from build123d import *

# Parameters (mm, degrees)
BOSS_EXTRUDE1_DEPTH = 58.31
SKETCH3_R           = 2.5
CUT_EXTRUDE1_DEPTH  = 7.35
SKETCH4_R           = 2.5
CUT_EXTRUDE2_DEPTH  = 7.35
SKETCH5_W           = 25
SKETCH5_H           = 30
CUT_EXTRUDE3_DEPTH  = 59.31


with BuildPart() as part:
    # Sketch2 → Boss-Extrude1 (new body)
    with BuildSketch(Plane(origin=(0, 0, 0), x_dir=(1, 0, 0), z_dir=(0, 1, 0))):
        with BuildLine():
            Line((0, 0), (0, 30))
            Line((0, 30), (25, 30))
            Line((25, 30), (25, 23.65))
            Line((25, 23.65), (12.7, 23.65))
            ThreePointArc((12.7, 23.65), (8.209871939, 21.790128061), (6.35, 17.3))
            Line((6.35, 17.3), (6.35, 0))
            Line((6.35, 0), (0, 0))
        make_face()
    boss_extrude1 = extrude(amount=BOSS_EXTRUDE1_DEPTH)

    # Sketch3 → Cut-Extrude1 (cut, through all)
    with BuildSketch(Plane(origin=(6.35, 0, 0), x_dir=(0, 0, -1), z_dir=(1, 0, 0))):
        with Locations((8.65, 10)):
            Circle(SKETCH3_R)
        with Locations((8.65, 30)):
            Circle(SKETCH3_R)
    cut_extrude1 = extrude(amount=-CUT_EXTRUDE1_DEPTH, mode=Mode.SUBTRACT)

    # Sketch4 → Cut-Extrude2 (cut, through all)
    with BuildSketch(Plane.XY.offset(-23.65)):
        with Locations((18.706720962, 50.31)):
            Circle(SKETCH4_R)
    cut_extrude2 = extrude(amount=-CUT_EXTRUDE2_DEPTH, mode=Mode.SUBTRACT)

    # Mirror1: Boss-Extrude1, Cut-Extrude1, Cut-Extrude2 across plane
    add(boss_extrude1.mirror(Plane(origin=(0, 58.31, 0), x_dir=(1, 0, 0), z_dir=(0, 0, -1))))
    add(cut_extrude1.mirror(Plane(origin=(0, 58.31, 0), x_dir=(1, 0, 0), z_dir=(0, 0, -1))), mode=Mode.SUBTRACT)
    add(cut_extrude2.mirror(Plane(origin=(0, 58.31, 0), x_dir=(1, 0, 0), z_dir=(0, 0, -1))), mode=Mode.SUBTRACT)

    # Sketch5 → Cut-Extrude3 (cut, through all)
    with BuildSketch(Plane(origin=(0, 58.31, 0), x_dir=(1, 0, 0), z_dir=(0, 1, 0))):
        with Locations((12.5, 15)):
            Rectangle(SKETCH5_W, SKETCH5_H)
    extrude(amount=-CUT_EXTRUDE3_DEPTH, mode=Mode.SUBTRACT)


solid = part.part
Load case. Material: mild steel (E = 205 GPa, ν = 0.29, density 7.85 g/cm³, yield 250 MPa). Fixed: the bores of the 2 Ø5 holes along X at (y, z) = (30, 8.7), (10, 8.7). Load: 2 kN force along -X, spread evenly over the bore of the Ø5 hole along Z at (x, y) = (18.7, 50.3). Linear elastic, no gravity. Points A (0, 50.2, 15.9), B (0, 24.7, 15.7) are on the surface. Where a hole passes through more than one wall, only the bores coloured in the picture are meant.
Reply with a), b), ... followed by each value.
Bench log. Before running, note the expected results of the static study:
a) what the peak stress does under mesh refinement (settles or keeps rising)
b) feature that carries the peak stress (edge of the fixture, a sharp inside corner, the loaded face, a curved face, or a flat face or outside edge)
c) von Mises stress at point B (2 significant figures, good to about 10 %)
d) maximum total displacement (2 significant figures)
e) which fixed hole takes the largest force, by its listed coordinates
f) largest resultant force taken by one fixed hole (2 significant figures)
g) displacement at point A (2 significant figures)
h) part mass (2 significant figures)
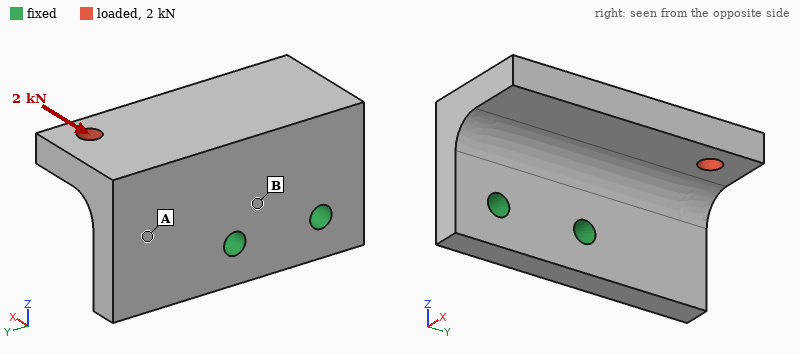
a) keeps rising
b) edge of the fixture
c) 100 MPa
d) 0.10 mm
e) (30, 8.7)
f) 3.1 kN
g) 0.036 mm
h) 140 g
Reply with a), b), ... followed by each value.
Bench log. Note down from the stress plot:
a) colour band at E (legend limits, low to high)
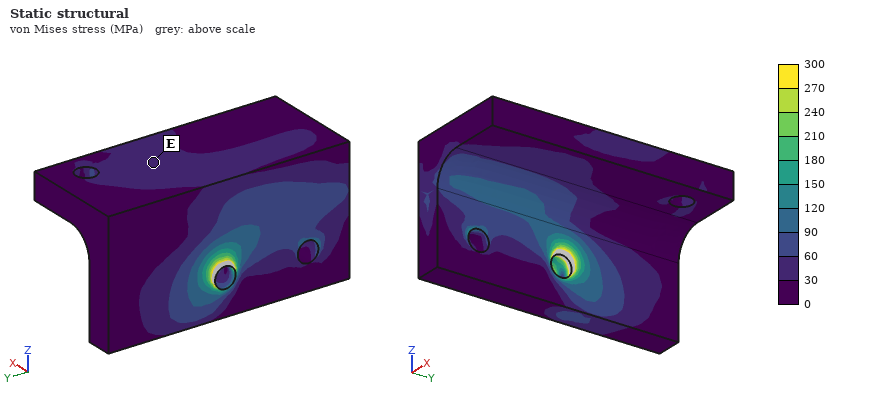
a) 30 to 60 MPa
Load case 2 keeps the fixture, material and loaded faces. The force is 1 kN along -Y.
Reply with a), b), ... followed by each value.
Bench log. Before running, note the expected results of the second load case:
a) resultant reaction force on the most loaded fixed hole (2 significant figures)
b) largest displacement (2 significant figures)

a) 1.0 kN
b) 17 µm
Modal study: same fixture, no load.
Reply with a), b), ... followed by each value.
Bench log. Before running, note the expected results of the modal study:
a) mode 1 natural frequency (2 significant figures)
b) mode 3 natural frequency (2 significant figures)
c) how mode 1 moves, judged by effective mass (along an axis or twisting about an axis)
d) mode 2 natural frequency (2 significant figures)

a) 3800 Hz
b) 9000 Hz
c) along X
d) 5600 Hz
